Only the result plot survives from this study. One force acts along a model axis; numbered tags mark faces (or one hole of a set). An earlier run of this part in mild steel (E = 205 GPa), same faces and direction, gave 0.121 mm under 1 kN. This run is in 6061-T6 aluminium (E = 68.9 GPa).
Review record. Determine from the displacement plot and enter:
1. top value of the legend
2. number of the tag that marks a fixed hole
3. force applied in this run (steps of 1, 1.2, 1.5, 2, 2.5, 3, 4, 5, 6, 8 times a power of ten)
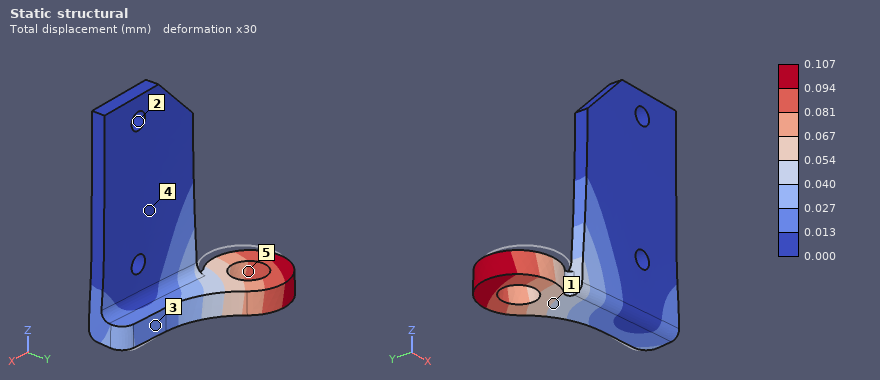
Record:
0.107 mm
2
300 N
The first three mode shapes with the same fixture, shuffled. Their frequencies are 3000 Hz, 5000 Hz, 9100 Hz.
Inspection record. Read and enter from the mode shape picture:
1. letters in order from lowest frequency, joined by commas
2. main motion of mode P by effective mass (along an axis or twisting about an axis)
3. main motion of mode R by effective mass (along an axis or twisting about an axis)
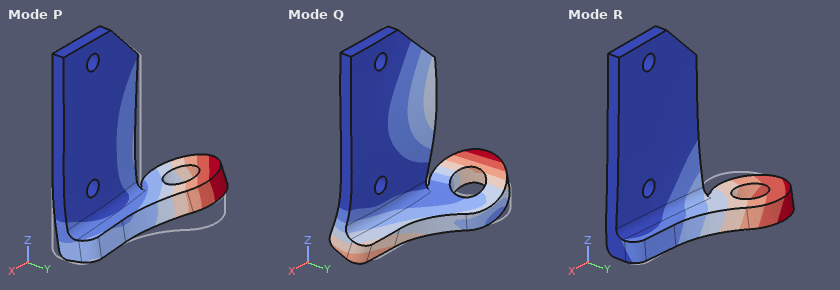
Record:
R, P, Q
along Z
along Y
